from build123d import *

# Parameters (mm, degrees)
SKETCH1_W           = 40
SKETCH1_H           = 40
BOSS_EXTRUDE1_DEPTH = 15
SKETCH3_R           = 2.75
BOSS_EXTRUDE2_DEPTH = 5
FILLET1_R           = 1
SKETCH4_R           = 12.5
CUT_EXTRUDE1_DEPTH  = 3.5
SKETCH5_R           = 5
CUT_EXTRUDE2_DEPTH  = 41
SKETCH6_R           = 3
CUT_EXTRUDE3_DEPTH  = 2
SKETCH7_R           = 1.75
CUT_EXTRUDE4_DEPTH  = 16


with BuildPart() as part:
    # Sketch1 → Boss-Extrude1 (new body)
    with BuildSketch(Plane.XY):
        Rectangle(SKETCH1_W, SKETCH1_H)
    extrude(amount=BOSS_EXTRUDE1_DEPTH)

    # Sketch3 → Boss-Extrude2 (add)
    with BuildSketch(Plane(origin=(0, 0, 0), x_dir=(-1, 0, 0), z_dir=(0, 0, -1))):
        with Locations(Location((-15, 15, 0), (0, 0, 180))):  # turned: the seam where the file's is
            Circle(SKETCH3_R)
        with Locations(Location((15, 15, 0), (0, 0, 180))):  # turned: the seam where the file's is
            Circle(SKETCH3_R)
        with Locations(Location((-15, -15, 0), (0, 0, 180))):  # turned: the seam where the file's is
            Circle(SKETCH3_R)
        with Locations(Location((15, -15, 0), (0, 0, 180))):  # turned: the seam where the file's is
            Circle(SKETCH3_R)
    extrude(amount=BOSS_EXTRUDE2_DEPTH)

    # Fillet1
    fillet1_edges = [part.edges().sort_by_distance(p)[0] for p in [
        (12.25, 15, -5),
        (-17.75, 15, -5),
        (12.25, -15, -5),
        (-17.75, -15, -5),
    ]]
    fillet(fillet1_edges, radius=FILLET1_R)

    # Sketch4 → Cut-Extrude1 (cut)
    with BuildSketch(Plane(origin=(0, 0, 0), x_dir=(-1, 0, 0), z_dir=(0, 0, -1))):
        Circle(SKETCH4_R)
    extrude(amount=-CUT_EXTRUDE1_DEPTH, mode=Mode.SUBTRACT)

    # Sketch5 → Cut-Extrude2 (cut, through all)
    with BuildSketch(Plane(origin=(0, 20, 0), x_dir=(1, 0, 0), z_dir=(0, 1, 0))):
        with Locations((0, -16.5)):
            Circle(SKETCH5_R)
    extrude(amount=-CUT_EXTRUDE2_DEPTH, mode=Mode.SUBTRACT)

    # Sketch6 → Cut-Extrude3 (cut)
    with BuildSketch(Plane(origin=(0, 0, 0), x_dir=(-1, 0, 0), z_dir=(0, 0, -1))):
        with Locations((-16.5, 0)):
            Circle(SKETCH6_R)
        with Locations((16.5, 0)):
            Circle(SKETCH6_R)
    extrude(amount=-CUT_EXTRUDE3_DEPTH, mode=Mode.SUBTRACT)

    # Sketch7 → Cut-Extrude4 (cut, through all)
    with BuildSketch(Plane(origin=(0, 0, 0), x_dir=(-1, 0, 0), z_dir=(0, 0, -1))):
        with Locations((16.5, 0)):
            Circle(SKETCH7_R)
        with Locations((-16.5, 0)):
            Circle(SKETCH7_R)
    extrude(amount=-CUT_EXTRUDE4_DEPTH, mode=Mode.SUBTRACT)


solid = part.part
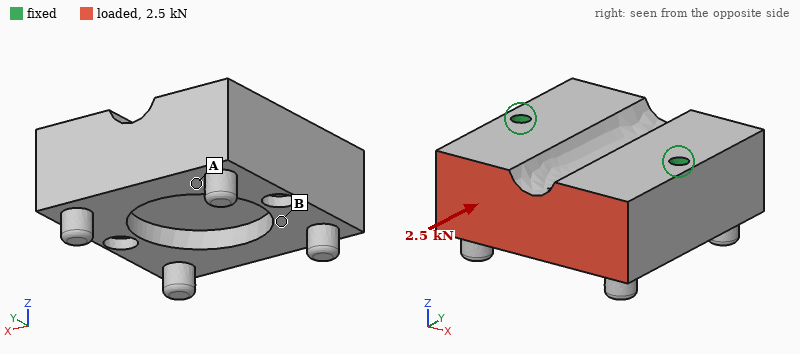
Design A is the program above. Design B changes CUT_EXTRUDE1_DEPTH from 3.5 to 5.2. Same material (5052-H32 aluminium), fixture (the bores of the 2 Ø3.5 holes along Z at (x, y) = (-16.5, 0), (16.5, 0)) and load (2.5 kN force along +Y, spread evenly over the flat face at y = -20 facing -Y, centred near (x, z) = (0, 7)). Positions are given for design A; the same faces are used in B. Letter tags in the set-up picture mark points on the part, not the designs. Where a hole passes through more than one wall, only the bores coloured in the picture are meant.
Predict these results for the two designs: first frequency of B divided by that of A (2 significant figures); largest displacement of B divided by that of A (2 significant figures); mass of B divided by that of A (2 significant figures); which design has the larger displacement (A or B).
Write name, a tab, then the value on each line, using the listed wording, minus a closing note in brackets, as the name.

first frequency of B divided by that of A	1.00
largest displacement of B divided by that of A	1.2
mass of B divided by that of A	0.96
which design has the larger displacement	B
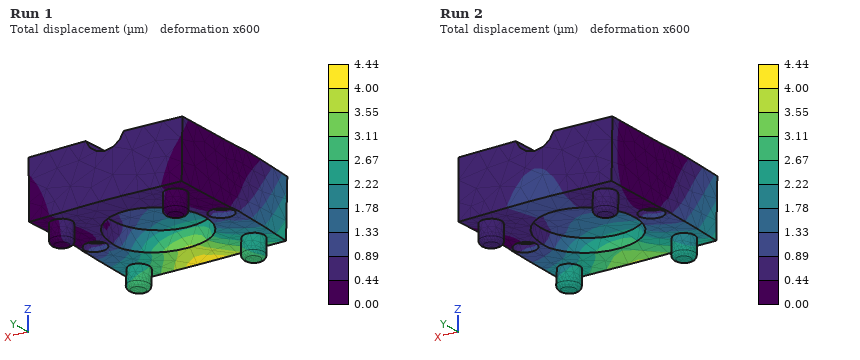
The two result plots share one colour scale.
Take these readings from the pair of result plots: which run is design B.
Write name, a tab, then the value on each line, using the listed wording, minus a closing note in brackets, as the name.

which run is design B	Run 1
